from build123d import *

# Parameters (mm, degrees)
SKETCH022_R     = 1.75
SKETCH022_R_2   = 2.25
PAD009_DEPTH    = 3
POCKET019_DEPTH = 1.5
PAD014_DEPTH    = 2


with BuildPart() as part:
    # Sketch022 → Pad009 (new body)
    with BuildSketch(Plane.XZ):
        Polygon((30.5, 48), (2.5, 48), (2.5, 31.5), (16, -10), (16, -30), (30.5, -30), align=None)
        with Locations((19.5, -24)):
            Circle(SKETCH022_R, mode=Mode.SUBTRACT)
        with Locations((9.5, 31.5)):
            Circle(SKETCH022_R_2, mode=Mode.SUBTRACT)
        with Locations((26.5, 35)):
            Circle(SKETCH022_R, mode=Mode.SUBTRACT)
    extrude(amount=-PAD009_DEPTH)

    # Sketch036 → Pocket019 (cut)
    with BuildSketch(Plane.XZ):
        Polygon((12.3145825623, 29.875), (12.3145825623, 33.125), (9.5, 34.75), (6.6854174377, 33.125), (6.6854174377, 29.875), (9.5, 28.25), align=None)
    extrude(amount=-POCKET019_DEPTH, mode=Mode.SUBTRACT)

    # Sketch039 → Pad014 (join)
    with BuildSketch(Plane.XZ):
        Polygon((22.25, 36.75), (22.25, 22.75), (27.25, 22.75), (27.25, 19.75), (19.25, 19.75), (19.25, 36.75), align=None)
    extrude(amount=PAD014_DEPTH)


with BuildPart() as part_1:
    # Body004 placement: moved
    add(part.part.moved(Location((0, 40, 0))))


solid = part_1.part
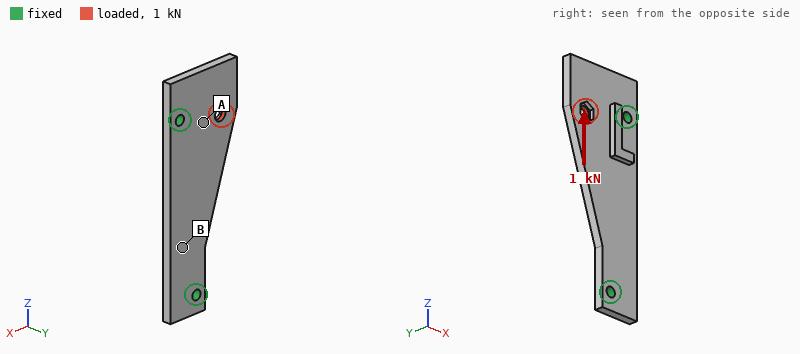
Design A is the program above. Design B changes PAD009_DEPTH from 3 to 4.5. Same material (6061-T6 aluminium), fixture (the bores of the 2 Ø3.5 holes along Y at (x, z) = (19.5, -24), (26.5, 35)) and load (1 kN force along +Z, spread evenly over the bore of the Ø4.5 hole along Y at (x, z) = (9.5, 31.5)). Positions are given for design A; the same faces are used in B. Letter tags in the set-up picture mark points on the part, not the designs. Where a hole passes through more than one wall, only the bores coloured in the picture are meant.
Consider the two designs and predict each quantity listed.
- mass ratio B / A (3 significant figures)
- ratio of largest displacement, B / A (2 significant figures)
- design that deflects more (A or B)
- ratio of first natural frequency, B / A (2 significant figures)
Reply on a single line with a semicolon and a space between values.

1.49; 0.56; A; 1.4
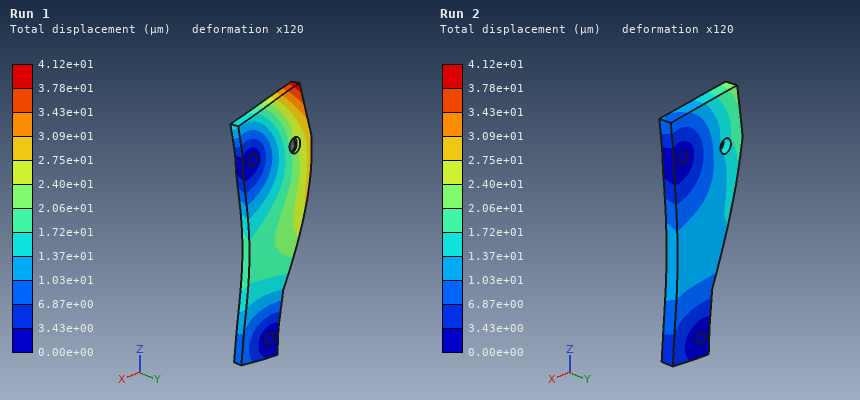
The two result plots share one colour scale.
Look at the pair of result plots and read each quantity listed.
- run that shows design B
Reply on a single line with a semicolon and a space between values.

Run 2
